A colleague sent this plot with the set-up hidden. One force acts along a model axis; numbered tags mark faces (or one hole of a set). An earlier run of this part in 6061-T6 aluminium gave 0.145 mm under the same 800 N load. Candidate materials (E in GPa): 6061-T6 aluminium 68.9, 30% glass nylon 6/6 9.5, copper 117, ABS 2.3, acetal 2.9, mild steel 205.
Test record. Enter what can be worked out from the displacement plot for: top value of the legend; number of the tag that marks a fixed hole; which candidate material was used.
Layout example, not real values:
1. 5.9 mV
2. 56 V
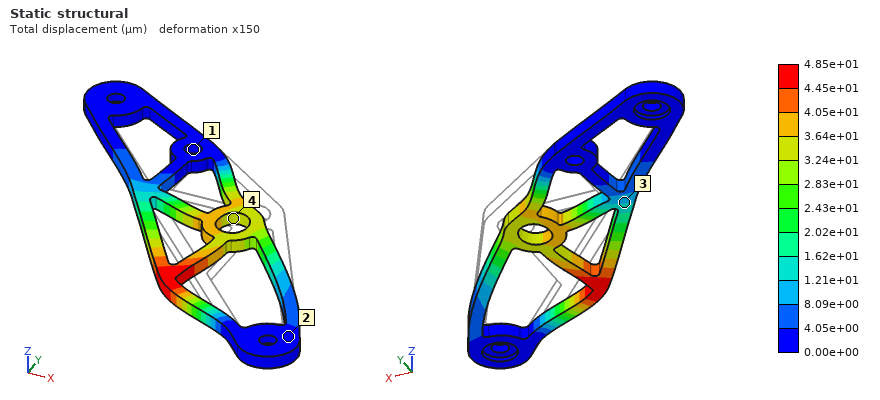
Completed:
1. 4.85e+01 µm
2. 1
3. mild steel
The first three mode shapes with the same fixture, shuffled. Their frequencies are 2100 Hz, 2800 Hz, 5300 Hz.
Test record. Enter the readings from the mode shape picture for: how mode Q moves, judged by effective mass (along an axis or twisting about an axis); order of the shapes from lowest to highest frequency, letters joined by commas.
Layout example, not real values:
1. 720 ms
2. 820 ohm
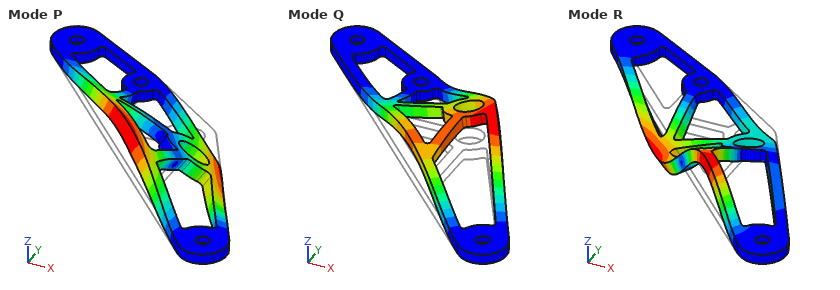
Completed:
1. along Z
2. Q, P, R
